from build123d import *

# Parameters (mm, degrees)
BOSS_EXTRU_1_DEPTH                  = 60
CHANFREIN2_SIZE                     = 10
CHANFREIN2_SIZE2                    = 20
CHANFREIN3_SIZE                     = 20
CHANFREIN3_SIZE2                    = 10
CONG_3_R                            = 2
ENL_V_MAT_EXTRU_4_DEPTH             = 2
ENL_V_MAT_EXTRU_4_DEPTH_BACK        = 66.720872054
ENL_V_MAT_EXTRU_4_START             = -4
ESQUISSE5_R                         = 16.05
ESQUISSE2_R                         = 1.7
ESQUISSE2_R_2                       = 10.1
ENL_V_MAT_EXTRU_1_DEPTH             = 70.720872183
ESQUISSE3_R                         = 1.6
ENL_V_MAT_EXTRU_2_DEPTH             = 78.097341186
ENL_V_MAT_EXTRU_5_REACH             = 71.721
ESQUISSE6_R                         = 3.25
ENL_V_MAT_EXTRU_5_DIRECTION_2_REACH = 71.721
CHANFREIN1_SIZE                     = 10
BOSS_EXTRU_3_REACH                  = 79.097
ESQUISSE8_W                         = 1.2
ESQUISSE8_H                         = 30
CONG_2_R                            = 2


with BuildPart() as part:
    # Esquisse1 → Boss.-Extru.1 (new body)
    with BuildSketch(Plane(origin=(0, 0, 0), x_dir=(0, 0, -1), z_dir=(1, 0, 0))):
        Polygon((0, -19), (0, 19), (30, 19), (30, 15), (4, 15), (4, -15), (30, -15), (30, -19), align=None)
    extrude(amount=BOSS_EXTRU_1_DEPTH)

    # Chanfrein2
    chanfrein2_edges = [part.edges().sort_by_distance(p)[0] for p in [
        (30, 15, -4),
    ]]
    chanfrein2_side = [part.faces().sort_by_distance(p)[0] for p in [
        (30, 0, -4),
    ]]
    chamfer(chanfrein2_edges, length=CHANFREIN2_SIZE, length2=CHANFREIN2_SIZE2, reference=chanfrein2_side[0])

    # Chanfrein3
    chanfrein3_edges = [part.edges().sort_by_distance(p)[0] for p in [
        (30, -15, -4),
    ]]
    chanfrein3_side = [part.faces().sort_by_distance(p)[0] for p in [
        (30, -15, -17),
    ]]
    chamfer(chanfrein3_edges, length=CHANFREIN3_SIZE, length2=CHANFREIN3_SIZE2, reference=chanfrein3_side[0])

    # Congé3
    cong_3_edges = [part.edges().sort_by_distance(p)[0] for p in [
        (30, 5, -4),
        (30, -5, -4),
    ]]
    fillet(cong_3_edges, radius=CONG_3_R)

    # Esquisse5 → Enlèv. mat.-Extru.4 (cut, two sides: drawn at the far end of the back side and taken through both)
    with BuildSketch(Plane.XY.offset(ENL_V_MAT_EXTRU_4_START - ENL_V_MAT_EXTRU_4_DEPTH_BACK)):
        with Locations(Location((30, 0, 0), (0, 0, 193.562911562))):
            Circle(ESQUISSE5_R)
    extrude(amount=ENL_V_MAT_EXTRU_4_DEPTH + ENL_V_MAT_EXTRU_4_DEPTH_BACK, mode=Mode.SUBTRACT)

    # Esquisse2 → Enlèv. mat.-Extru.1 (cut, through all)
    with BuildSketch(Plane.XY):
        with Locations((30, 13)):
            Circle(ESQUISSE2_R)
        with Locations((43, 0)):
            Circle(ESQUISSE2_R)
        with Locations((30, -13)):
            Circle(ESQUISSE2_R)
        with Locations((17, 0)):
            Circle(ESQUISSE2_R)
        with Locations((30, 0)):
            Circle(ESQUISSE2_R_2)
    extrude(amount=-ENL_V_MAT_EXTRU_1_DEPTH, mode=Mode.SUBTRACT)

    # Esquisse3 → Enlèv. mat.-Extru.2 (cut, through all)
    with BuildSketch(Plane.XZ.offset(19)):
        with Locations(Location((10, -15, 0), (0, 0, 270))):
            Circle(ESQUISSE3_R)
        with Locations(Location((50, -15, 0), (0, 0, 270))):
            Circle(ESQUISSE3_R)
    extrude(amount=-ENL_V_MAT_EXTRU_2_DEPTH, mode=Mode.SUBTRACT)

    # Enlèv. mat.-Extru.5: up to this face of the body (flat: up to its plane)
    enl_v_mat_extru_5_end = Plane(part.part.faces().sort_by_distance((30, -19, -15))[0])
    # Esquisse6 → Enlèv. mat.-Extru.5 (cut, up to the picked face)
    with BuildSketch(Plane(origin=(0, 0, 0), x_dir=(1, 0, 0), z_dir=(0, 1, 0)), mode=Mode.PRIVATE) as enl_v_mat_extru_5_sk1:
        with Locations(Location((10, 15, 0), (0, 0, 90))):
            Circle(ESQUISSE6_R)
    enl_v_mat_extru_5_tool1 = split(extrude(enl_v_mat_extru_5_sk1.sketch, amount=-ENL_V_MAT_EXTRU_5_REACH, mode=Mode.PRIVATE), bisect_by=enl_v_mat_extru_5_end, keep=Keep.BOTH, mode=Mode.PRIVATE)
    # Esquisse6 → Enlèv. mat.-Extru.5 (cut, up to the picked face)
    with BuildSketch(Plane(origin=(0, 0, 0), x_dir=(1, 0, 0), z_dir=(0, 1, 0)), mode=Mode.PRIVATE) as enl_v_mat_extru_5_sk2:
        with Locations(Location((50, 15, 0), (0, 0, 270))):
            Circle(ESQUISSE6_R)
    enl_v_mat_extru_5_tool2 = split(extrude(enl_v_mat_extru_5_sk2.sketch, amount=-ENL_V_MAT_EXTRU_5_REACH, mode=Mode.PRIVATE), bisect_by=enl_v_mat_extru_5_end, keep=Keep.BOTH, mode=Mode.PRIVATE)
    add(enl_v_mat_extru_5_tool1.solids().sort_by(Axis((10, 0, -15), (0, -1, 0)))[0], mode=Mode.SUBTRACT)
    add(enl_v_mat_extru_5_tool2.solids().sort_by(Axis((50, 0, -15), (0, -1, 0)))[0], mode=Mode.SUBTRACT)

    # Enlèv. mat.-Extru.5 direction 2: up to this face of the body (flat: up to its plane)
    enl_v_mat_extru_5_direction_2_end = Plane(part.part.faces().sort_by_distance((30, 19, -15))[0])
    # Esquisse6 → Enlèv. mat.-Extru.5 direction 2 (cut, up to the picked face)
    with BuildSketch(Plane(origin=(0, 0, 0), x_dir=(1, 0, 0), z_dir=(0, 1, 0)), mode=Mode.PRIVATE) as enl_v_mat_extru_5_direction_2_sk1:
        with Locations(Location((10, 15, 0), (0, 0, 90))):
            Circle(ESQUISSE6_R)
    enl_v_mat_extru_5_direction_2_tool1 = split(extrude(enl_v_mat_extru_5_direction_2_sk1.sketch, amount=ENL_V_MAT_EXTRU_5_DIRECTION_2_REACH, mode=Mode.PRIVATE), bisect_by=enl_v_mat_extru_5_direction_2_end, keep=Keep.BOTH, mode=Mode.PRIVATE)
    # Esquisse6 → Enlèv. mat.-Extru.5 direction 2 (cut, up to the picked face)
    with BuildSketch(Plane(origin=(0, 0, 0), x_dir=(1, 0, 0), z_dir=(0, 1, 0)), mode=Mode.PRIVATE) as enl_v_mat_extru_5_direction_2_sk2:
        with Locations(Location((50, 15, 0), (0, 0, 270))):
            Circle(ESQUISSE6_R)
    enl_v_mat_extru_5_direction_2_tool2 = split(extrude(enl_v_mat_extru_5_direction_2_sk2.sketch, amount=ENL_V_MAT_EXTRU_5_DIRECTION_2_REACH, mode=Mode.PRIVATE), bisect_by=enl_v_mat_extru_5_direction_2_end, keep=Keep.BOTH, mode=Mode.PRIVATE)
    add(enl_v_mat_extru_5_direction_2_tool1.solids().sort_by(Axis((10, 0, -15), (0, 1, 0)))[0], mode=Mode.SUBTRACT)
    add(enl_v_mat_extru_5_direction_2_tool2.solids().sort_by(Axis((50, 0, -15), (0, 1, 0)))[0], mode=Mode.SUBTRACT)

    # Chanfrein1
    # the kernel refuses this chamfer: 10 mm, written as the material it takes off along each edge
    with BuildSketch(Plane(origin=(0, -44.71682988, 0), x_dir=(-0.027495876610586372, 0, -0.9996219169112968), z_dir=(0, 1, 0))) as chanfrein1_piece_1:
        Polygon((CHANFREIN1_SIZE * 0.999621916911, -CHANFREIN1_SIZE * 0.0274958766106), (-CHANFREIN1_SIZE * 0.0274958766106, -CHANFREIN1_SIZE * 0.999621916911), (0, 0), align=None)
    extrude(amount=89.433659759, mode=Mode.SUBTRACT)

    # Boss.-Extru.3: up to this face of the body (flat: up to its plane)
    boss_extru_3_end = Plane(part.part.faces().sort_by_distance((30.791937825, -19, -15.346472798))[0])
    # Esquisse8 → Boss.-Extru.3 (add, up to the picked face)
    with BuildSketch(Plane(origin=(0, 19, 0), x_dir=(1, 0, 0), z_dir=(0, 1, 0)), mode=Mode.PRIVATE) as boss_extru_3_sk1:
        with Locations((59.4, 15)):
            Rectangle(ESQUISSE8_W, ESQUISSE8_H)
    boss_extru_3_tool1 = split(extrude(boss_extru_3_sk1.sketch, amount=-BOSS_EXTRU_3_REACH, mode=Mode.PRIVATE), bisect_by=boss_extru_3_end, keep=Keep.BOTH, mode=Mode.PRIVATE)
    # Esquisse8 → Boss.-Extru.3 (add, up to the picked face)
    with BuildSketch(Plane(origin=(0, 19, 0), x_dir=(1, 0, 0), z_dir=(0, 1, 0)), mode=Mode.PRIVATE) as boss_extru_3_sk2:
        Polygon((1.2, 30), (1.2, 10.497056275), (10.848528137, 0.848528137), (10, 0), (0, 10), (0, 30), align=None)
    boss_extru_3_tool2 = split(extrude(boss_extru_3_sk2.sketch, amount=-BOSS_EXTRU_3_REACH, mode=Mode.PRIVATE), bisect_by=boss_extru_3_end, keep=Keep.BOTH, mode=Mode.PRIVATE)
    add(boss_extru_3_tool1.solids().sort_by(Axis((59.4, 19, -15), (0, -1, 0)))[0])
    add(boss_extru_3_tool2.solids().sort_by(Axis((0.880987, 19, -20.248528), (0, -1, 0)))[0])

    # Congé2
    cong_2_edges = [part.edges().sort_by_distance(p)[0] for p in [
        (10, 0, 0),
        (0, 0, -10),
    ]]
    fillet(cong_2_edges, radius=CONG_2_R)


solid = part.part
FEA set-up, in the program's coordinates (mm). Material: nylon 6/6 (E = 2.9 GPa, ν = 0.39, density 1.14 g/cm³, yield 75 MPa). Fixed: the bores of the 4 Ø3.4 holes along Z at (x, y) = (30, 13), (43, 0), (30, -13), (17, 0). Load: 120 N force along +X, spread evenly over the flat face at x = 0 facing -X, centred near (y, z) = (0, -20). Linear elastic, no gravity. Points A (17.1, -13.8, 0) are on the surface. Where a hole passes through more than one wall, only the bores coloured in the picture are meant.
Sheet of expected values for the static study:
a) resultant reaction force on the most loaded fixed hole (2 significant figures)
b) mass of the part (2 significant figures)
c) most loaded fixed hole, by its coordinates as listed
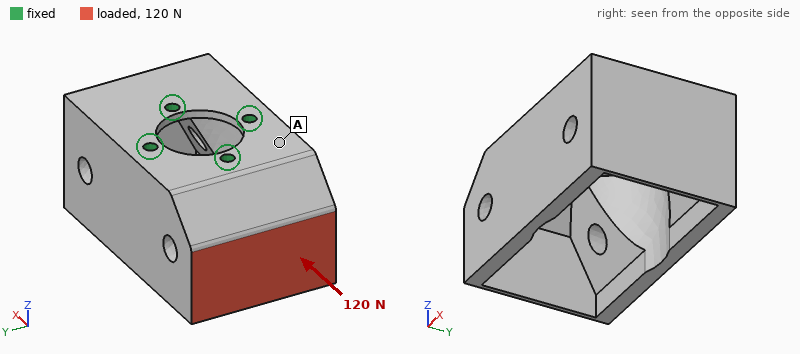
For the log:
76 N
29 g
(17, 0)
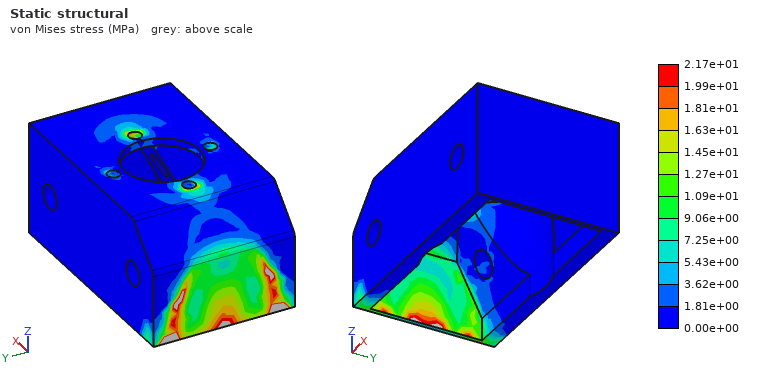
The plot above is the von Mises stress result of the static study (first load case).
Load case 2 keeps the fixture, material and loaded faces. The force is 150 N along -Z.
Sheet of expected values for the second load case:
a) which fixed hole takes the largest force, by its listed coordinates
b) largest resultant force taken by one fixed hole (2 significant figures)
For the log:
(17, 0)
190 N
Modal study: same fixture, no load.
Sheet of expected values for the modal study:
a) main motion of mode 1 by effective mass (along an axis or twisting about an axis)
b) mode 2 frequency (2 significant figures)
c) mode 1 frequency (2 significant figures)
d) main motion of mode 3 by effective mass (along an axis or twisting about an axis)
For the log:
along X
1200 Hz
1100 Hz
along Y
